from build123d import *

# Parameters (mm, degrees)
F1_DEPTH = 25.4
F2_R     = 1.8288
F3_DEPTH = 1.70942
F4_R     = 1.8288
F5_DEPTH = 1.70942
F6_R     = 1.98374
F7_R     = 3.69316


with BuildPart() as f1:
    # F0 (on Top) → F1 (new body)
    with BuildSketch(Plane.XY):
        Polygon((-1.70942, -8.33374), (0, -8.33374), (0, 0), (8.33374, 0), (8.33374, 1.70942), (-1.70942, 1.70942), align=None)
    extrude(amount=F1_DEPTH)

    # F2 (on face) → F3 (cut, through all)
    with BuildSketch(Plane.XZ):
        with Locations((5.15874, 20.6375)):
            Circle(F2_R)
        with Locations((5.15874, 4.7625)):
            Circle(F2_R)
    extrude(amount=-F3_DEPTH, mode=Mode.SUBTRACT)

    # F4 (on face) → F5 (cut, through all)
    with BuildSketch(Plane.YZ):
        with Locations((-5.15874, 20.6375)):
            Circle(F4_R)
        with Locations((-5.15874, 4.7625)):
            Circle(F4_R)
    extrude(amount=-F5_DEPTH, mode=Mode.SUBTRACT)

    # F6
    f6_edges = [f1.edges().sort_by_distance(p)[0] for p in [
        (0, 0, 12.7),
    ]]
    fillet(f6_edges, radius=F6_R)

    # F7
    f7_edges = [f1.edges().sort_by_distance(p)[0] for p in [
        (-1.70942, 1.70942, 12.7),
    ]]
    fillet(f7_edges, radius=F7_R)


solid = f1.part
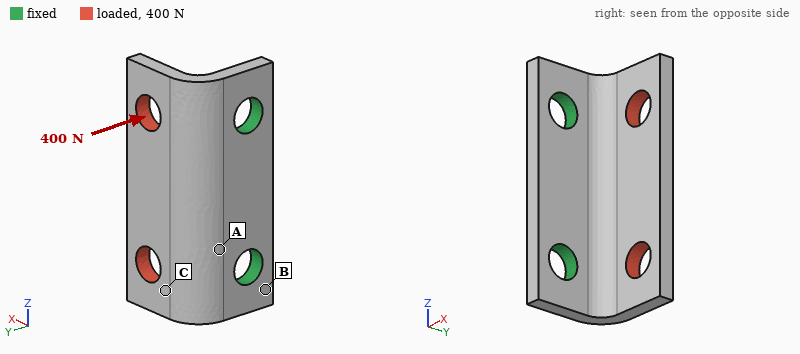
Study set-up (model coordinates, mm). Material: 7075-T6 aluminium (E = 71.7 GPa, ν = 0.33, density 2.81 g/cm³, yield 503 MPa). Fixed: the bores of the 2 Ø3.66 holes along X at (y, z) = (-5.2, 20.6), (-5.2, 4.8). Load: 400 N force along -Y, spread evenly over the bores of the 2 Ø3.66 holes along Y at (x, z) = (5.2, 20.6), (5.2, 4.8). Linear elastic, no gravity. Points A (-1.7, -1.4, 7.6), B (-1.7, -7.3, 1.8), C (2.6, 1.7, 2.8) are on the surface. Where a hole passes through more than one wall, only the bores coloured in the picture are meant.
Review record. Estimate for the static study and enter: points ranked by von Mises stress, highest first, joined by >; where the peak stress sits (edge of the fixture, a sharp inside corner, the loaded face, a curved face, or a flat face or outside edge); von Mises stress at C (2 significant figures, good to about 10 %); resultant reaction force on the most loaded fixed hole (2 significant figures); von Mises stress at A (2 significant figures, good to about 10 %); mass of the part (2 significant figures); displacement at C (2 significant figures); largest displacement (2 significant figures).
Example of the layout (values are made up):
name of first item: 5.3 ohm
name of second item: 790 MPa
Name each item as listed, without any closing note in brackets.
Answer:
points ranked by von Mises stress, highest first, joined by >: A > C > B
where the peak stress sits: a flat face or outside edge
von Mises stress at C: 86 MPa
resultant reaction force on the most loaded fixed hole: 200 N
von Mises stress at A: 140 MPa
mass of the part: 1.9 g
displacement at C: 0.082 mm
largest displacement: 0.19 mm
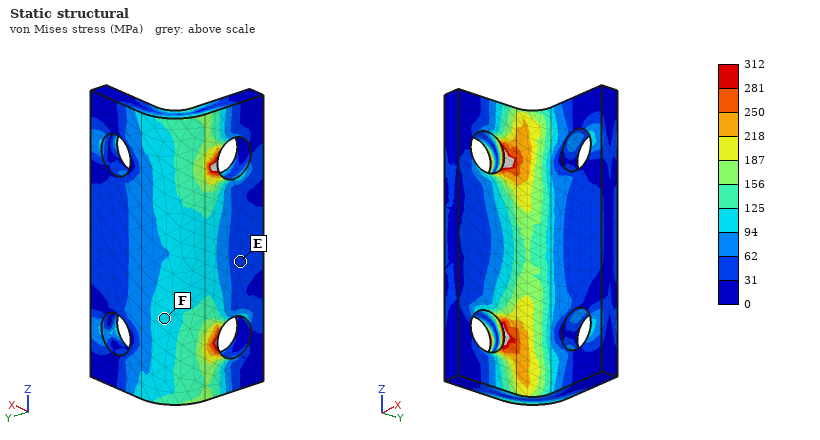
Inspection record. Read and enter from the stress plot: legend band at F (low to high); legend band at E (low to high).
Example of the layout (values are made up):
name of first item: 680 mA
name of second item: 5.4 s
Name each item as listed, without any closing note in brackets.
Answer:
legend band at F: 94 to 125 MPa
legend band at E: 31 to 62 MPa
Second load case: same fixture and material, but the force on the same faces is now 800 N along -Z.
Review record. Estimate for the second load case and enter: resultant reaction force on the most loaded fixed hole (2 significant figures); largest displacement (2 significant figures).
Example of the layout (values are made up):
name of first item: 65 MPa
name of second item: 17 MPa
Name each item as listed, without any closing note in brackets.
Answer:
resultant reaction force on the most loaded fixed hole: 530 N
largest displacement: 73 µm
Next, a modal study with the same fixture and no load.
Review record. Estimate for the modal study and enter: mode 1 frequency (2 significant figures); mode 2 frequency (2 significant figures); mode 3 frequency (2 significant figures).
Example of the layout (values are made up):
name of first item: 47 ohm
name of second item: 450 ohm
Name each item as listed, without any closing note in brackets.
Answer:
mode 1 frequency: 9900 Hz
mode 2 frequency: 15 kHz
mode 3 frequency: 28 kHz
